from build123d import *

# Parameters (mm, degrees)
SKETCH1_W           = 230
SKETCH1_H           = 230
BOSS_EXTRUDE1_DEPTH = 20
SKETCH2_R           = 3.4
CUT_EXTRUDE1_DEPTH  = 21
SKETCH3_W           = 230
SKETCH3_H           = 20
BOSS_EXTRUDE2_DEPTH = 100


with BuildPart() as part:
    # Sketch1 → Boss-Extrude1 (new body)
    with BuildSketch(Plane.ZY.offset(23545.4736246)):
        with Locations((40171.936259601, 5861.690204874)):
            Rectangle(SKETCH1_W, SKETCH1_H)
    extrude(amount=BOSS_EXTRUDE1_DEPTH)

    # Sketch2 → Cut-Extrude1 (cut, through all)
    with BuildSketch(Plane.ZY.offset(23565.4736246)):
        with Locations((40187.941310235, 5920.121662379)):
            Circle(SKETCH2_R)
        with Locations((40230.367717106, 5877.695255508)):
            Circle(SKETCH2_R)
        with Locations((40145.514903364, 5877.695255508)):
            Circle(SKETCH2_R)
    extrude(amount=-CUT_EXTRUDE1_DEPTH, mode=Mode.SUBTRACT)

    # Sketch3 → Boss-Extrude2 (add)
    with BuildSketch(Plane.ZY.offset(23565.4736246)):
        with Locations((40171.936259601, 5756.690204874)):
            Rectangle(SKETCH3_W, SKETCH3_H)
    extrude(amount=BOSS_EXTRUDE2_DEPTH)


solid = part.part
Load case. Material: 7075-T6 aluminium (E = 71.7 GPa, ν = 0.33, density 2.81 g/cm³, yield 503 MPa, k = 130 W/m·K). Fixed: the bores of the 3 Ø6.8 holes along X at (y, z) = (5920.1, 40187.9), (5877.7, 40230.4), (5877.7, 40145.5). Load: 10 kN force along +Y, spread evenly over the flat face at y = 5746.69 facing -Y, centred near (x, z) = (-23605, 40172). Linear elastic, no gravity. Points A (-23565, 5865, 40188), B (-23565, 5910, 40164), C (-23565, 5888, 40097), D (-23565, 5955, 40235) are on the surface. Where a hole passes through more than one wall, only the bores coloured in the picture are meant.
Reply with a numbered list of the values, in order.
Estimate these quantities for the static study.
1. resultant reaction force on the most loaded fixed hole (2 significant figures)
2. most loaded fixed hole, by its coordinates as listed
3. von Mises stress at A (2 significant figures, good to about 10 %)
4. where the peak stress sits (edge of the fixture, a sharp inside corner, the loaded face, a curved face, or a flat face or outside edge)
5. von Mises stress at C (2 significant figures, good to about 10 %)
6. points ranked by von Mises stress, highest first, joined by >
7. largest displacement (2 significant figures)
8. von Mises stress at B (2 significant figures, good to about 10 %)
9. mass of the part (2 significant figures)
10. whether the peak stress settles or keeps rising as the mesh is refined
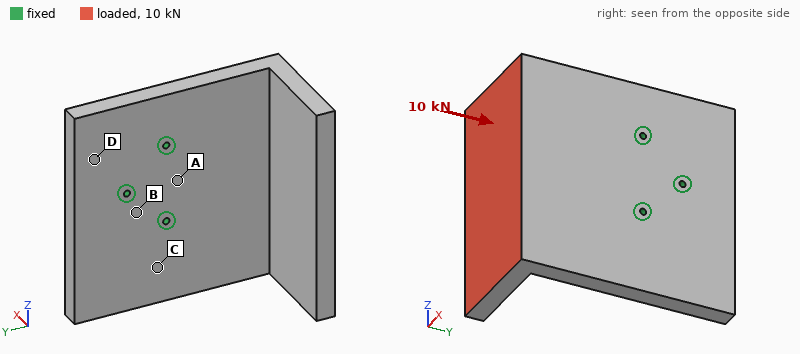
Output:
1. 6.0 kN
2. (5877.7, 40145.5)
3. 30 MPa
4. edge of the fixture
5. 18 MPa
6. A > C > B > D
7. 0.90 mm
8. 8.5 MPa
9. 4.3 kg
10. keeps rising
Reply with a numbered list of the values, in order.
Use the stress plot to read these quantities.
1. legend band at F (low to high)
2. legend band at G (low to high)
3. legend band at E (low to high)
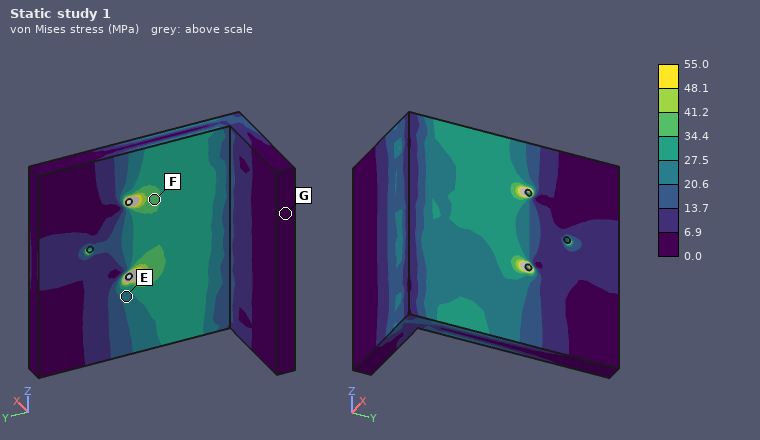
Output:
1. 34.4 to 41.2 MPa
2. 0.0 to 6.9 MPa
3. 20.6 to 27.5 MPa
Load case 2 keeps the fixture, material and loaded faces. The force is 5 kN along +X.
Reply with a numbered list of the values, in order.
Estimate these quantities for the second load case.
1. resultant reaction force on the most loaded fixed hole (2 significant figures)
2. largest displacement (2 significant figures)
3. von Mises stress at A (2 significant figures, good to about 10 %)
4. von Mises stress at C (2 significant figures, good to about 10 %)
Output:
1. 6.3 kN
2. 0.72 mm
3. 34 MPa
4. 21 MPa
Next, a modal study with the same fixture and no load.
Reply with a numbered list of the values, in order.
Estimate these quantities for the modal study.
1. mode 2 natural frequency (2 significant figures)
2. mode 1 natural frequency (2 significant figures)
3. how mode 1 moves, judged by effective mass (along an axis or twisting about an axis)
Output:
1. 590 Hz
2. 360 Hz
3. along X
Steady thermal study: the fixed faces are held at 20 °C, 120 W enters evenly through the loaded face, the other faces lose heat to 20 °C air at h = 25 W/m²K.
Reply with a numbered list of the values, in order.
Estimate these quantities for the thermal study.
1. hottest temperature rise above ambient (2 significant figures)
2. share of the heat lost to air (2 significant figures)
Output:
1. 28 K
2. 36 %
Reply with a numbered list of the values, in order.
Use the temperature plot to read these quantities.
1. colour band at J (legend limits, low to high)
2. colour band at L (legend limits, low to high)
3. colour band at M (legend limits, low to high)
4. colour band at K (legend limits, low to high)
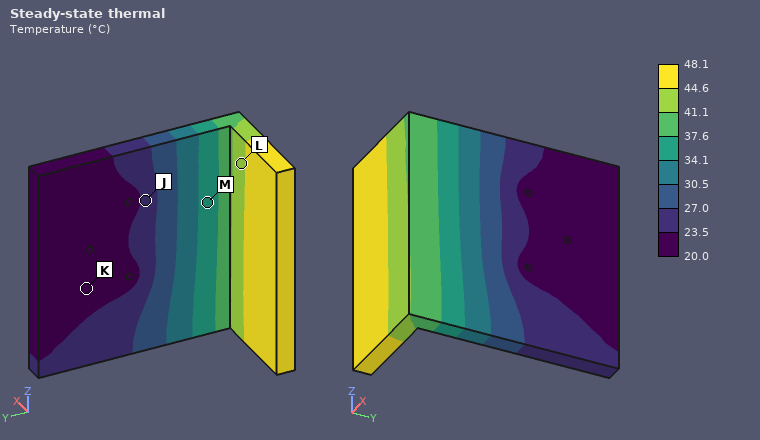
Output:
1. 23.5 to 27.0 °C
2. 41.1 to 44.6 °C
3. 34.1 to 37.6 °C
4. 20.0 to 23.5 °C
